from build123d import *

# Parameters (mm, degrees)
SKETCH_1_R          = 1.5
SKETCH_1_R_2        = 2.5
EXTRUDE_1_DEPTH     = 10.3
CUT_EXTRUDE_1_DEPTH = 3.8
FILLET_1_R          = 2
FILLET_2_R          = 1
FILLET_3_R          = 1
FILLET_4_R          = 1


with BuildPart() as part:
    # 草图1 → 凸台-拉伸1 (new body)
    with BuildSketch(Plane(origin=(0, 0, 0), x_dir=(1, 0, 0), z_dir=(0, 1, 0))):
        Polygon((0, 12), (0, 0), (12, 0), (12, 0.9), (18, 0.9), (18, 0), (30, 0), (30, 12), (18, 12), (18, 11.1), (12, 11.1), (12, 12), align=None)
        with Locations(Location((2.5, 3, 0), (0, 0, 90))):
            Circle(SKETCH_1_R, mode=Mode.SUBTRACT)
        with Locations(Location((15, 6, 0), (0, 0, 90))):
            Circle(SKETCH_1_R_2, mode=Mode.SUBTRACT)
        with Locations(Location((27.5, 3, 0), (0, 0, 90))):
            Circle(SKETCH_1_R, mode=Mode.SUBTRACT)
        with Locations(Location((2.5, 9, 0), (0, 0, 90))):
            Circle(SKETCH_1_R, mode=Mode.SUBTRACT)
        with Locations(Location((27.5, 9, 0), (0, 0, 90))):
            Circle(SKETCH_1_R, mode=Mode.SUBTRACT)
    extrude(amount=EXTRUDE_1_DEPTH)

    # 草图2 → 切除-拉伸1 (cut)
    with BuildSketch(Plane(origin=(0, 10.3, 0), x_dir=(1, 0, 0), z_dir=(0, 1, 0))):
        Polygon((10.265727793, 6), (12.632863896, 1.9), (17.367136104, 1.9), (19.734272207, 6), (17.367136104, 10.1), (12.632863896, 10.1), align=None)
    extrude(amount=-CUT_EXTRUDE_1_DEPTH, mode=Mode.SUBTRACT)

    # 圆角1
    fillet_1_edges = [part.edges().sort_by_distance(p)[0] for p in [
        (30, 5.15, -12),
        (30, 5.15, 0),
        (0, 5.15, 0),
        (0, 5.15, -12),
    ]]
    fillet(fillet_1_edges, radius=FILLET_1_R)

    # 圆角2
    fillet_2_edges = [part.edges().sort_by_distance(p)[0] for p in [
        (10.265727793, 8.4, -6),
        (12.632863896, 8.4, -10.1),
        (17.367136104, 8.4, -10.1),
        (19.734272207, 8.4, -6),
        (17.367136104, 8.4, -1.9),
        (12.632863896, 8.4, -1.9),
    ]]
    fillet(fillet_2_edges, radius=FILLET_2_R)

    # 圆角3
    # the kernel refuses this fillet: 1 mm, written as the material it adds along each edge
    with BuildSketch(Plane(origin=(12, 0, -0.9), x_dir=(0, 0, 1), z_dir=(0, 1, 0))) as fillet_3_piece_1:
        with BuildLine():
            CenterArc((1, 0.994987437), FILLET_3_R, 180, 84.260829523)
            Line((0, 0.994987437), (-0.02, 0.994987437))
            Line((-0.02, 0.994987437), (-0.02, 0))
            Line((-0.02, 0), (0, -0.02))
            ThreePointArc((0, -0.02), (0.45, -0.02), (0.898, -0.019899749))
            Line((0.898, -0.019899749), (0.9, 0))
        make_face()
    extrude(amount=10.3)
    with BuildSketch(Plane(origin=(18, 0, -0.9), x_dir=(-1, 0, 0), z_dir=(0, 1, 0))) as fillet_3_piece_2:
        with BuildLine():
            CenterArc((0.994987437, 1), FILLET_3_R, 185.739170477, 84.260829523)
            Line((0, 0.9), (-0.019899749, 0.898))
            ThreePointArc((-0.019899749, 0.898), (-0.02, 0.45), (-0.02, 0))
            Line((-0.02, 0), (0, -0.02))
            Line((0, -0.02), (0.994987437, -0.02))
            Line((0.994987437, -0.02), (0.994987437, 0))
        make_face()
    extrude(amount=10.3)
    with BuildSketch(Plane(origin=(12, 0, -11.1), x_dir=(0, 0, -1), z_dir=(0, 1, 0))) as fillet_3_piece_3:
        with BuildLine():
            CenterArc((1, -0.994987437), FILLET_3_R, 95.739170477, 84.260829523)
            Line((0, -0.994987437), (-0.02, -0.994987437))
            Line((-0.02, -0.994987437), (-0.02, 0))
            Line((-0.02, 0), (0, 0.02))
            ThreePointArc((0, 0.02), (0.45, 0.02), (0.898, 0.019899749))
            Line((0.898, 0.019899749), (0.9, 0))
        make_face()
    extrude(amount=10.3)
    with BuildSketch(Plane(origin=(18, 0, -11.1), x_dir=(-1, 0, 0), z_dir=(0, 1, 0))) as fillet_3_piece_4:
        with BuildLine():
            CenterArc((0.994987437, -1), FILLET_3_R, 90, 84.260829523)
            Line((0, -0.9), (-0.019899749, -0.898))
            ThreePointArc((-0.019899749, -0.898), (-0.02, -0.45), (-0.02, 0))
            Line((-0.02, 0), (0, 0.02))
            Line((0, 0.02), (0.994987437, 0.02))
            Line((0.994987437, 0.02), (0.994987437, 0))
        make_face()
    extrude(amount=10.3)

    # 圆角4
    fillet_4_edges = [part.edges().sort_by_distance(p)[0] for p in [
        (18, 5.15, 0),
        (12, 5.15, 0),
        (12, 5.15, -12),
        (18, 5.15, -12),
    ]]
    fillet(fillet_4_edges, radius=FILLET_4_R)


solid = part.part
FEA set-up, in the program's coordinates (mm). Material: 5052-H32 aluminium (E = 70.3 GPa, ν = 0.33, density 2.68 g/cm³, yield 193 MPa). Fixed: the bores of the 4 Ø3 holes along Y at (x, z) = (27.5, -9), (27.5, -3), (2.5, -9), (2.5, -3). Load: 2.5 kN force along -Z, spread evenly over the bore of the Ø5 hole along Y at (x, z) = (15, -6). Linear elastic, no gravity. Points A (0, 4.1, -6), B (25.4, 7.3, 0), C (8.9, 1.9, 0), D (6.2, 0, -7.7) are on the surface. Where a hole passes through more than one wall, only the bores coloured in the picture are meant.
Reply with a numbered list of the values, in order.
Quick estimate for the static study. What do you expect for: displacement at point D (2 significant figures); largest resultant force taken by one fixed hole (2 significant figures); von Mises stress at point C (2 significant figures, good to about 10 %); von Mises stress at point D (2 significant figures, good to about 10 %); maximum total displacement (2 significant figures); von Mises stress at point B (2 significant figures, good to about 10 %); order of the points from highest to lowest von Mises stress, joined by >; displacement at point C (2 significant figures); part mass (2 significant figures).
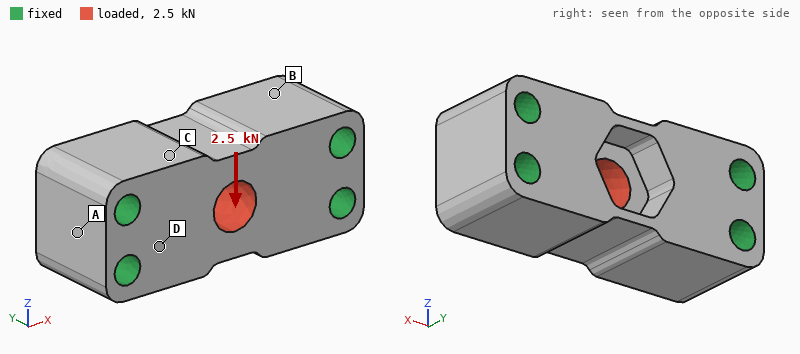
1. 2.0 µm
2. 1.2 kN
3. 13 MPa
4. 38 MPa
5. 11 µm
6. 23 MPa
7. D > B > C > A
8. 5.3 µm
9. 7.8 g
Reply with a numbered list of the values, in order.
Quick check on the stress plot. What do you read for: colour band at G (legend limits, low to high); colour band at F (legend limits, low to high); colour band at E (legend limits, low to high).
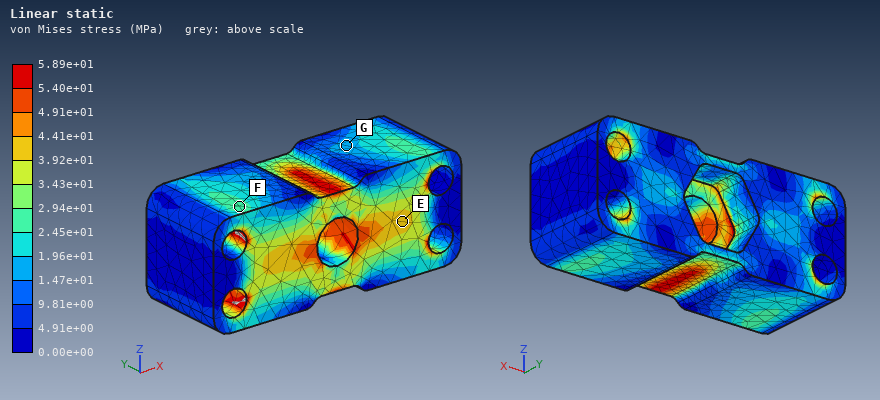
1. 1.47e+01 to 1.96e+01 MPa
2. 2.45e+01 to 2.94e+01 MPa
3. 3.92e+01 to 4.41e+01 MPa
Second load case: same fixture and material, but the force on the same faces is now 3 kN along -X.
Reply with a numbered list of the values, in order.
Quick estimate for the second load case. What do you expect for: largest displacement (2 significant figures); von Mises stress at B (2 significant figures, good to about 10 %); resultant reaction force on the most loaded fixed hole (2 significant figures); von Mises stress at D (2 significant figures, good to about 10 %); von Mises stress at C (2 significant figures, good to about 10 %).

1. 3.3 µm
2. 7.4 MPa
3. 770 N
4. 20 MPa
5. 9.7 MPa
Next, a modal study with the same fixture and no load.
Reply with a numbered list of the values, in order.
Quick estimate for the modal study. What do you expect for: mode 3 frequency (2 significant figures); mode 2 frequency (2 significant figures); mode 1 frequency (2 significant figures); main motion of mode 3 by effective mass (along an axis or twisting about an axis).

1. 73 kHz
2. 61 kHz
3. 60 kHz
4. twisting about X
